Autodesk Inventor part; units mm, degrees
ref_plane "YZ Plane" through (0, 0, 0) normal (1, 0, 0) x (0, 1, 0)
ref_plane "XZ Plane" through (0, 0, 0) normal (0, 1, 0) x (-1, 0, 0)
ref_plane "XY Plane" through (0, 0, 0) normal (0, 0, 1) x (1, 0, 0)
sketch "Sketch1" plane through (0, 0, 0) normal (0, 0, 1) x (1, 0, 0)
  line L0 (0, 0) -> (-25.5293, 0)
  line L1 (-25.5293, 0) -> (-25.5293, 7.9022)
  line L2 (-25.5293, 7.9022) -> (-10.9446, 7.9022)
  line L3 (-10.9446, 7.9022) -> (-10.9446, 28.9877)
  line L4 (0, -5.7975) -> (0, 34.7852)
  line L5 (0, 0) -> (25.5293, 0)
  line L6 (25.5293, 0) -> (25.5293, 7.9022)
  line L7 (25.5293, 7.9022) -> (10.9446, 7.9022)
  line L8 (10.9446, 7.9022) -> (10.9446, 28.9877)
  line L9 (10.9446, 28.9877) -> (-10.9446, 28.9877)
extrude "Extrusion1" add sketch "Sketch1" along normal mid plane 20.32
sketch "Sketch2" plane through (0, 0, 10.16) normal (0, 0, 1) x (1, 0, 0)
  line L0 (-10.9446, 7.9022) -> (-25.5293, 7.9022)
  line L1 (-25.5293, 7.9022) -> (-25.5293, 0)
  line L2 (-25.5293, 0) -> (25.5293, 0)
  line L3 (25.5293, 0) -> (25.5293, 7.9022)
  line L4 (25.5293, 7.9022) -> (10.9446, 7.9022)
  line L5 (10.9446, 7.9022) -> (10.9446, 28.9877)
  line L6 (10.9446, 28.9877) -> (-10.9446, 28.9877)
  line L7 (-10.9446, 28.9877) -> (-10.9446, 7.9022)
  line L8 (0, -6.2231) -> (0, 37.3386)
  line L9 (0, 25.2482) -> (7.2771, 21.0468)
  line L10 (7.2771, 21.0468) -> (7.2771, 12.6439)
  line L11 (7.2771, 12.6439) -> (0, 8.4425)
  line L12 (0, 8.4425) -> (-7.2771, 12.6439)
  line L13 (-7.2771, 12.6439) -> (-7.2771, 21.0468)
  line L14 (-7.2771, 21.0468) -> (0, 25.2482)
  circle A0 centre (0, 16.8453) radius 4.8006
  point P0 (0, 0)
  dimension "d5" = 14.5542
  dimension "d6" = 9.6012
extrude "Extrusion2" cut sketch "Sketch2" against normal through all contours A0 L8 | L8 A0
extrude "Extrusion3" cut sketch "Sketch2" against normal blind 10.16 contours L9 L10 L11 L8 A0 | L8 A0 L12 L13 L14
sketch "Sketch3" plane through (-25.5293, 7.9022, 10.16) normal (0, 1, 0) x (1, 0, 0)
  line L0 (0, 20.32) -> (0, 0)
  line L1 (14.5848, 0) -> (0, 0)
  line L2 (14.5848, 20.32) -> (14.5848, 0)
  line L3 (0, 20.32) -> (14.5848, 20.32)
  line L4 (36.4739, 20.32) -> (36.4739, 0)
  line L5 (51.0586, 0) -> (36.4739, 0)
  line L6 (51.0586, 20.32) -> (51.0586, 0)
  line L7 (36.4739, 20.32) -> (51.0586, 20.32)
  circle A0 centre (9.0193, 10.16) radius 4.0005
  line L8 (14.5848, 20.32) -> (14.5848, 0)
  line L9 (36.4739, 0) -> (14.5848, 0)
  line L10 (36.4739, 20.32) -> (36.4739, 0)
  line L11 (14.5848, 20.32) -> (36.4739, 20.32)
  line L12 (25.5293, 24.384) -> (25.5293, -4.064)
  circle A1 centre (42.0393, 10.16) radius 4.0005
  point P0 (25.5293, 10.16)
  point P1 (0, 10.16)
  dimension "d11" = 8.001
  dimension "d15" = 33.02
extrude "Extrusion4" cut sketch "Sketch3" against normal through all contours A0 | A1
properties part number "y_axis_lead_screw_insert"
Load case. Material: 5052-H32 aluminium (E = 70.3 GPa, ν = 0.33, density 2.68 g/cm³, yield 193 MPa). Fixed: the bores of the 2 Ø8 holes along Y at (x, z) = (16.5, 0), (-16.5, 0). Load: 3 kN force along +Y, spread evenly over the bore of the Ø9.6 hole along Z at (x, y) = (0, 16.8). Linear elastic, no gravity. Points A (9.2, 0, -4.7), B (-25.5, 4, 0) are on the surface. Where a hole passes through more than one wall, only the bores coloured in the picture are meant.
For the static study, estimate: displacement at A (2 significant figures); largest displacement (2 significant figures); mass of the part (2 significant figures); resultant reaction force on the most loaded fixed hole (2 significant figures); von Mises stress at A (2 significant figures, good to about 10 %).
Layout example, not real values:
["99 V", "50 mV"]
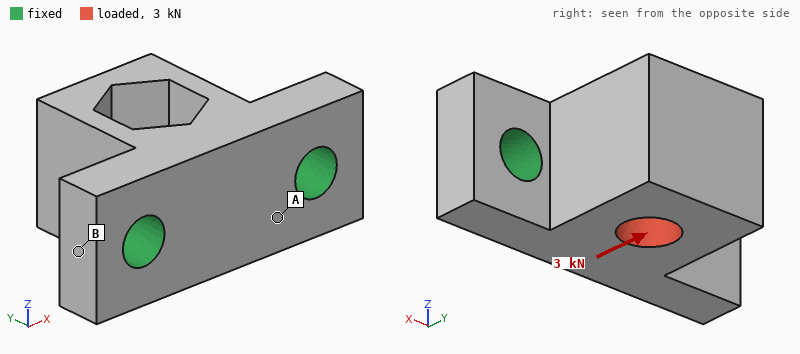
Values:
["5.0 µm", "20 µm", "38 g", "1.6 kN", "14 MPa"]
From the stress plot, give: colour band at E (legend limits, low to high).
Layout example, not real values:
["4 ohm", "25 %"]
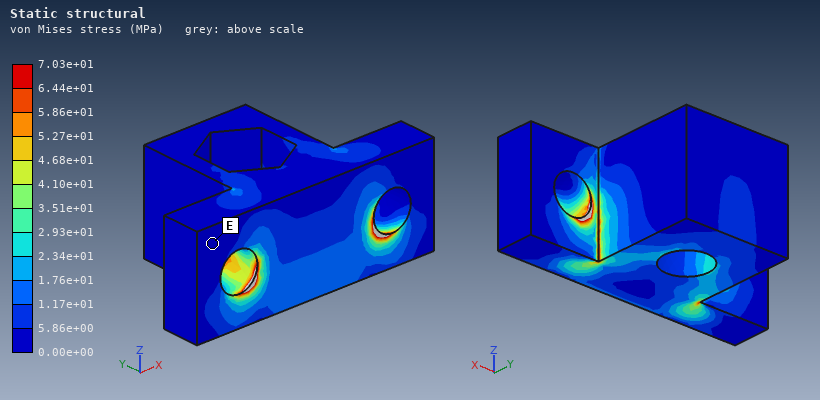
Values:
["0.00e+00 to 5.86e+00 MPa"]
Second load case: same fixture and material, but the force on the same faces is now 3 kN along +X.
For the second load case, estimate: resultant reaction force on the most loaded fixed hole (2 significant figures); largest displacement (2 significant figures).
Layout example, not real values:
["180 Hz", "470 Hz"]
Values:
["2.1 kN", "21 µm"]
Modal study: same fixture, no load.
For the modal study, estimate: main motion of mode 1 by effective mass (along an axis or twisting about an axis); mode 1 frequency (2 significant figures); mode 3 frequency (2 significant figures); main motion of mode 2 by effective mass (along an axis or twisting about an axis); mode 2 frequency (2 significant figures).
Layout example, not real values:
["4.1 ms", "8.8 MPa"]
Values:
["along Z", "9600 Hz", "22 kHz", "along X", "14 kHz"]
